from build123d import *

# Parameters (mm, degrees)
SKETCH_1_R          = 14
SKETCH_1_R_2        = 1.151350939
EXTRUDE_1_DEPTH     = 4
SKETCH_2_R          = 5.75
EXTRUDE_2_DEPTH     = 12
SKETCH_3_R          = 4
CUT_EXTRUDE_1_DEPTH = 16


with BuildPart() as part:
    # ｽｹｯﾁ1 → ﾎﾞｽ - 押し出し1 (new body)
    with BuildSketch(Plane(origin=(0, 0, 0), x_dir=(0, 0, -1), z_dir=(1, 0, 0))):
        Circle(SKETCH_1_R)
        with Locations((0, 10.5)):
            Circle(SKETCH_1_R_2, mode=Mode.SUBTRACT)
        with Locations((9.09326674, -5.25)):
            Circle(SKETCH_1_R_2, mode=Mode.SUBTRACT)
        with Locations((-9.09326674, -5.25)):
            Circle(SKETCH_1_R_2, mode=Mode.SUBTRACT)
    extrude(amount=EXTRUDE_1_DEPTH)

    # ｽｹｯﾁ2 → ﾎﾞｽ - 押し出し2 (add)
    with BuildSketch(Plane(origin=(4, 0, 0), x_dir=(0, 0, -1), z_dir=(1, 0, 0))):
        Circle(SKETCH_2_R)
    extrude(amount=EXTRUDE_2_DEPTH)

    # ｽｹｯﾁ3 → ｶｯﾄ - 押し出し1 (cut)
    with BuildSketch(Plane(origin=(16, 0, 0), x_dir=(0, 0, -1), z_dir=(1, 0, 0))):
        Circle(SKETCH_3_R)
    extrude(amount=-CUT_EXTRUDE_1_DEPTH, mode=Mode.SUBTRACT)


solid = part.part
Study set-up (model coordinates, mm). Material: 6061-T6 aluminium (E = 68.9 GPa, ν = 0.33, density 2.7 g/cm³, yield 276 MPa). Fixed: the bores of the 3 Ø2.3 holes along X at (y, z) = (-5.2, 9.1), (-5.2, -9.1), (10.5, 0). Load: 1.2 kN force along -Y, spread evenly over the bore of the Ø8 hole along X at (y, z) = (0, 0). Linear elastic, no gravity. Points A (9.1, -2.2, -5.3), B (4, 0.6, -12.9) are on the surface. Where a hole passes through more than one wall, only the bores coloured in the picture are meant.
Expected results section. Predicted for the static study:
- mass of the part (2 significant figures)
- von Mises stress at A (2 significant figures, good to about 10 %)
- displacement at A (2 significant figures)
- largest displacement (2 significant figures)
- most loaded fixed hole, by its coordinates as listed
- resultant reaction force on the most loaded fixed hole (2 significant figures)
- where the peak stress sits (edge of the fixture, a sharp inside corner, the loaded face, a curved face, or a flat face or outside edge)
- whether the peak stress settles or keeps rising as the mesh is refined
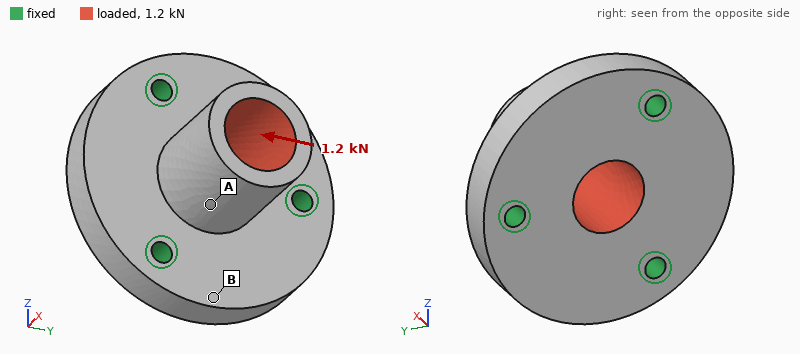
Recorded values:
7.7 g
25 MPa
13 µm
27 µm
(10.5, 0)
620 N
edge of the fixture
keeps rising
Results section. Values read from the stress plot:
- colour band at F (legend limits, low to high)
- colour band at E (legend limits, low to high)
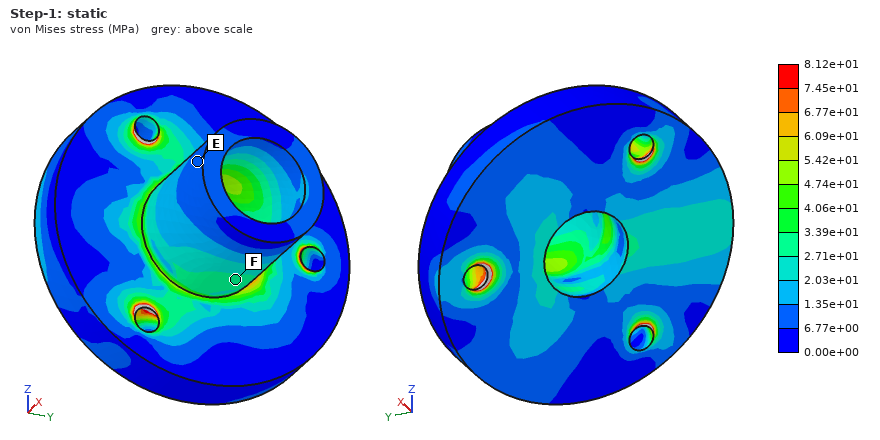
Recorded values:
2.71e+01 to 3.39e+01 MPa
6.77e+00 to 1.35e+01 MPa
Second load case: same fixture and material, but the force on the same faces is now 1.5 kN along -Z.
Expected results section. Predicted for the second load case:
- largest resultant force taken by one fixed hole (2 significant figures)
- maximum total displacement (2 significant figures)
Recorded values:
710 N
34 µm
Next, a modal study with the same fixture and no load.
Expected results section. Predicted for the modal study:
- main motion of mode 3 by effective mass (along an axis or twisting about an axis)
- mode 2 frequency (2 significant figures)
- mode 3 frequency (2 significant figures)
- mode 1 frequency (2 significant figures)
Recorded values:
along X
24 kHz
34 kHz
24 kHz
